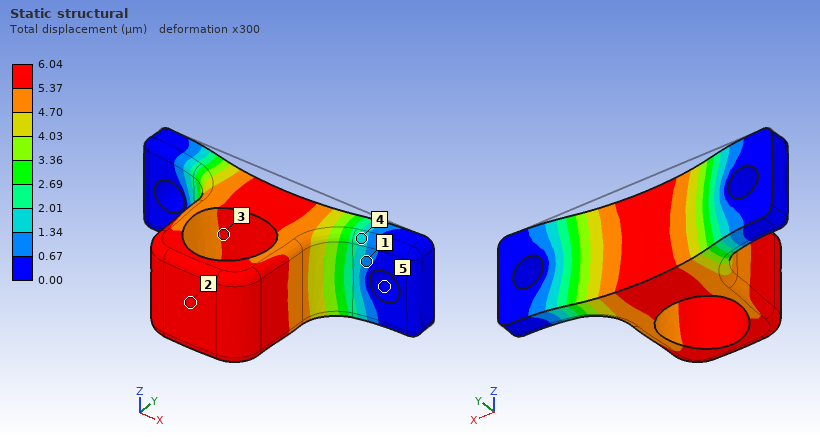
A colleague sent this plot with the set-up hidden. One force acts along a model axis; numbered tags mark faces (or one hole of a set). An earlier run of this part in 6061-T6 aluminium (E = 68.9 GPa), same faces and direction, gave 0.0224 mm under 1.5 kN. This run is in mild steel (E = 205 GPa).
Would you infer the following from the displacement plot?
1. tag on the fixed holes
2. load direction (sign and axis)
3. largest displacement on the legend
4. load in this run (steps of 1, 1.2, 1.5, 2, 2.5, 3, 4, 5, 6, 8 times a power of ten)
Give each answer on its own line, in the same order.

5
-Y
6.04 µm
1.2 kN
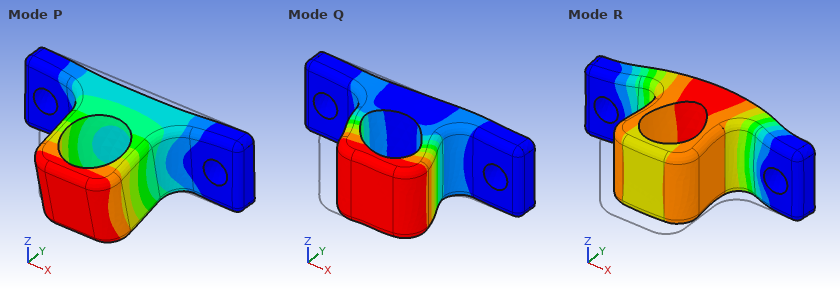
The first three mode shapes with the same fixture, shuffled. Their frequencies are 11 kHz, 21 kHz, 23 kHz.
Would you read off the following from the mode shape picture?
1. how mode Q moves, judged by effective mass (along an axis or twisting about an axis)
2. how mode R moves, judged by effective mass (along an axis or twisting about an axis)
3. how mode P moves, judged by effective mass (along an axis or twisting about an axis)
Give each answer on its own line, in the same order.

along X
along Y
along Z
